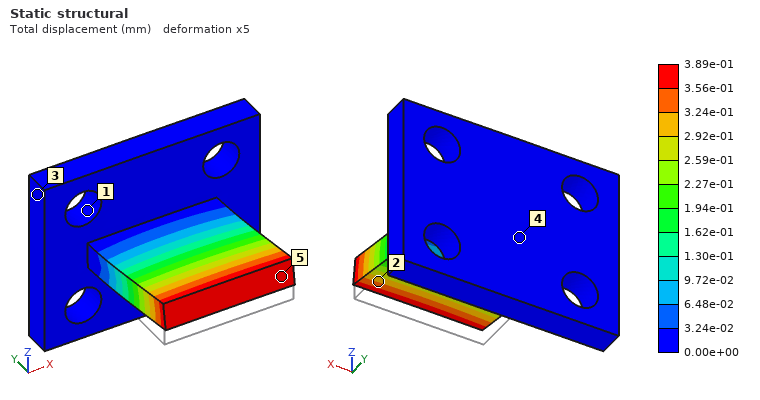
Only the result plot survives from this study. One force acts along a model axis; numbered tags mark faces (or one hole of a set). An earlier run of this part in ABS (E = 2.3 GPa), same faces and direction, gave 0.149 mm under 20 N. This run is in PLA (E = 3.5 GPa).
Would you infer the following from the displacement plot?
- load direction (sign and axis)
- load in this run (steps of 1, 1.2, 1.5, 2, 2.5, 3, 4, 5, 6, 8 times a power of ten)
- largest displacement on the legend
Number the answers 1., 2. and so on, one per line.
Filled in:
1. +Z
2. 80 N
3. 3.89e-01 mm
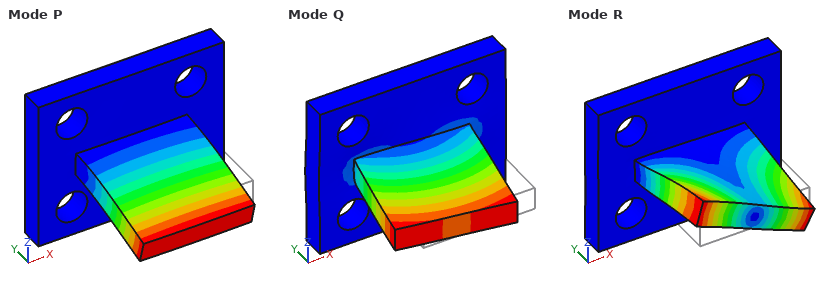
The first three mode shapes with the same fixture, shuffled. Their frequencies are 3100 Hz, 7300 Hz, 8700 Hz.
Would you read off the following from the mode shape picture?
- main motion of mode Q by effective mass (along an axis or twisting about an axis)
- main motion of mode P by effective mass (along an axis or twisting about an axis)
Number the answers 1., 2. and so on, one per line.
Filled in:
1. along X
2. along Z
